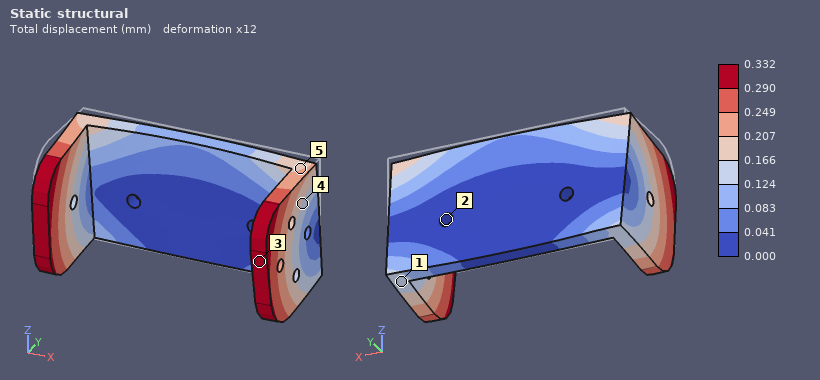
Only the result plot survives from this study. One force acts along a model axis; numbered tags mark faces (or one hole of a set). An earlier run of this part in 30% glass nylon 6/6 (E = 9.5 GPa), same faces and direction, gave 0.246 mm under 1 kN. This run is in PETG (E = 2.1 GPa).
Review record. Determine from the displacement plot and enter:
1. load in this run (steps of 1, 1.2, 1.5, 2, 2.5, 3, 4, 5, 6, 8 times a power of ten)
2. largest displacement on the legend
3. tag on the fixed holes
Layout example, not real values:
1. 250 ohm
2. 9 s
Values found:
1. 300 N
2. 0.332 mm
3. 2
